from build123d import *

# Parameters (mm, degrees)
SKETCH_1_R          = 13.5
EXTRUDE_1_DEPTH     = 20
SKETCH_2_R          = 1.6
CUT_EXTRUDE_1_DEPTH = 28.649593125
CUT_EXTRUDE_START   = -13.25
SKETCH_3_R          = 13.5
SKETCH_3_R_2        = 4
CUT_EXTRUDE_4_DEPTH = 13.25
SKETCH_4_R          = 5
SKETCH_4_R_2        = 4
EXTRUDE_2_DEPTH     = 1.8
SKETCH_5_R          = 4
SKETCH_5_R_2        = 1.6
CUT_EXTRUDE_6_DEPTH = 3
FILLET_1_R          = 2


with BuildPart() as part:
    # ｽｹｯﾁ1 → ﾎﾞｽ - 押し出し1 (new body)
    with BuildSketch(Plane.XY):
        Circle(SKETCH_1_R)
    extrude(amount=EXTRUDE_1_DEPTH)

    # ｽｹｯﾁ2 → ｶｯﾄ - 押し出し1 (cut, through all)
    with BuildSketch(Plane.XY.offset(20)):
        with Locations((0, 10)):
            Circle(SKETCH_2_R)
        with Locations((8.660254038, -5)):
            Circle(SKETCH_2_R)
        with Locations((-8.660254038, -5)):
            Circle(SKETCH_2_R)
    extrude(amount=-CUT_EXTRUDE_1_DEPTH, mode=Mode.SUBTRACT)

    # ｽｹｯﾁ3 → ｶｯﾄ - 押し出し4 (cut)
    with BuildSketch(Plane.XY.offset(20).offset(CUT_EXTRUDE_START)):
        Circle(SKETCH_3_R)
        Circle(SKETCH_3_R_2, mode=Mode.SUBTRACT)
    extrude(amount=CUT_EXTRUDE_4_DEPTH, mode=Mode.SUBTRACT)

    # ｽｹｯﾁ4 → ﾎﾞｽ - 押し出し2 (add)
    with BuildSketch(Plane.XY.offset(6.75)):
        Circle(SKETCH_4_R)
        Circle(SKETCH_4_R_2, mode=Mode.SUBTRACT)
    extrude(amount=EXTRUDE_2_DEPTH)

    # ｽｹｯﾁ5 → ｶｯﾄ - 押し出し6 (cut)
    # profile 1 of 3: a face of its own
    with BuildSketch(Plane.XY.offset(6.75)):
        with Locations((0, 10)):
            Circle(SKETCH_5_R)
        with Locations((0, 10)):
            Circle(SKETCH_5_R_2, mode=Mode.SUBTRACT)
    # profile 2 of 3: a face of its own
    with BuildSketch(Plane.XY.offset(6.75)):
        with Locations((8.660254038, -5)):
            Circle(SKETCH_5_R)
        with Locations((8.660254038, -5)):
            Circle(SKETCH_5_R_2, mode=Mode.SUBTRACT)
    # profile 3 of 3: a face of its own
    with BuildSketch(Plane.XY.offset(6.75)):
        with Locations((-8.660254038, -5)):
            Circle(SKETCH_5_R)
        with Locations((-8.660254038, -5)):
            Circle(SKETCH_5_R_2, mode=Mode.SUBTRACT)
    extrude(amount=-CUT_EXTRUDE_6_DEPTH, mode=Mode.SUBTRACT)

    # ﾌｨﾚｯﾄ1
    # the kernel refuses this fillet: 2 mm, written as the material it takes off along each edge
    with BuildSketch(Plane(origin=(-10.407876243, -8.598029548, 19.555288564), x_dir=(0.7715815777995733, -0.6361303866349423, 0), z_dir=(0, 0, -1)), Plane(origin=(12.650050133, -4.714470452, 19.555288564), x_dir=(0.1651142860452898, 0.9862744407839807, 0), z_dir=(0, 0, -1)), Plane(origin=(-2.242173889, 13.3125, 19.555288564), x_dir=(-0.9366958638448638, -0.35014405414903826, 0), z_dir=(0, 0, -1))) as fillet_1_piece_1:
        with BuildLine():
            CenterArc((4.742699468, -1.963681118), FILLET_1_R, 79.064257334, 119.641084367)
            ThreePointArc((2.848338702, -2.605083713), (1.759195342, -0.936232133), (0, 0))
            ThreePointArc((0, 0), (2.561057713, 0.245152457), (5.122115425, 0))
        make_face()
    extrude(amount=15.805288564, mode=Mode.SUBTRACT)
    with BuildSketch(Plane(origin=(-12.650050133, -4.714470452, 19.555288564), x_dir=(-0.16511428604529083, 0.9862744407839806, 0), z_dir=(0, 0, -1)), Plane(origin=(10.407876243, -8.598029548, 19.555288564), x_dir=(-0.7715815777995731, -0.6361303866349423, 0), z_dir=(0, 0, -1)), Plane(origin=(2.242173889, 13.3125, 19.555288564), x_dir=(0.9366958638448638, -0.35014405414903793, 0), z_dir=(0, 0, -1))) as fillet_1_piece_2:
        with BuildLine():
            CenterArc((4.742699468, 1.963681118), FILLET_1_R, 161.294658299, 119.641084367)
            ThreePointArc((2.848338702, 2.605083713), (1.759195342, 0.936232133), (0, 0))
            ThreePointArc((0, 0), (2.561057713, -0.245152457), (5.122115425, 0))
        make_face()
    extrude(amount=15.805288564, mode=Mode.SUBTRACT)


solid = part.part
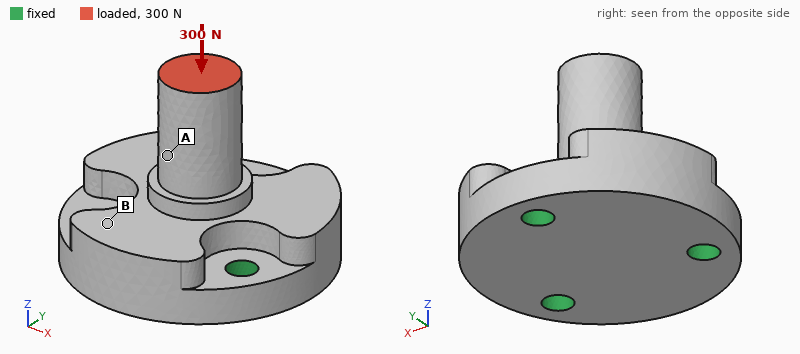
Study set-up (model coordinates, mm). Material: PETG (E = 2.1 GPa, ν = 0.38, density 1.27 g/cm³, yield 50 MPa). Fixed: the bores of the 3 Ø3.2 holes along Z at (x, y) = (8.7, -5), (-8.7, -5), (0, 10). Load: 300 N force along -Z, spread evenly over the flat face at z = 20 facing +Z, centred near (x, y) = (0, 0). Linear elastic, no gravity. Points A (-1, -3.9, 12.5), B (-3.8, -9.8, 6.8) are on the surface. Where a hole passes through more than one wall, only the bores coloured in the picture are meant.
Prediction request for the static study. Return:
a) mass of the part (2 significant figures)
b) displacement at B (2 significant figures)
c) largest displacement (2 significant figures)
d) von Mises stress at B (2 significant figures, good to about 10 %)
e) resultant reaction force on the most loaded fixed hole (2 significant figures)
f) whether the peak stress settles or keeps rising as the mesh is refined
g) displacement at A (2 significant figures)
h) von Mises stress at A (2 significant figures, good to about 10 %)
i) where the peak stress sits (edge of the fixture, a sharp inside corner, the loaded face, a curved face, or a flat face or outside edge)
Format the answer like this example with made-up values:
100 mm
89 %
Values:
5.1 g
13 µm
62 µm
1.2 MPa
110 N
keeps rising
41 µm
5.8 MPa
edge of the fixture
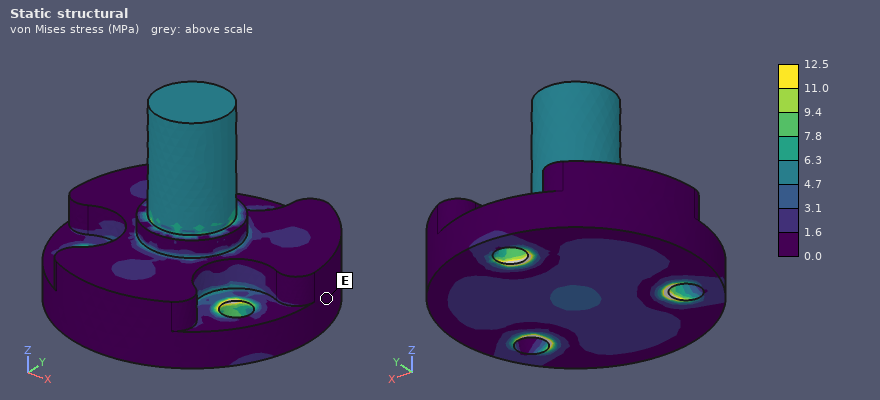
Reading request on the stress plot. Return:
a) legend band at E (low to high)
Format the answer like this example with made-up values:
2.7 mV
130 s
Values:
0.0 to 1.6 MPa
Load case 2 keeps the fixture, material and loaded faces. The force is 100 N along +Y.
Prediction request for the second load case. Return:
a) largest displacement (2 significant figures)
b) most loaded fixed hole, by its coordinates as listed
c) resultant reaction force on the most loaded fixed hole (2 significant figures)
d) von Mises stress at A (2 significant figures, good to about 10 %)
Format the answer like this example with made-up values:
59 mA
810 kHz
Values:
0.30 mm
(0, 10)
120 N
14 MPa
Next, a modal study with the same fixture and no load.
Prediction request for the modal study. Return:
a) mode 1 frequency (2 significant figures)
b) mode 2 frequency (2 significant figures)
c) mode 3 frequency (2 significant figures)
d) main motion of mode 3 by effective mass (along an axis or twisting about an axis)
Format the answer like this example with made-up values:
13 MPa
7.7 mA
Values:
5500 Hz
5500 Hz
9500 Hz
along Z
